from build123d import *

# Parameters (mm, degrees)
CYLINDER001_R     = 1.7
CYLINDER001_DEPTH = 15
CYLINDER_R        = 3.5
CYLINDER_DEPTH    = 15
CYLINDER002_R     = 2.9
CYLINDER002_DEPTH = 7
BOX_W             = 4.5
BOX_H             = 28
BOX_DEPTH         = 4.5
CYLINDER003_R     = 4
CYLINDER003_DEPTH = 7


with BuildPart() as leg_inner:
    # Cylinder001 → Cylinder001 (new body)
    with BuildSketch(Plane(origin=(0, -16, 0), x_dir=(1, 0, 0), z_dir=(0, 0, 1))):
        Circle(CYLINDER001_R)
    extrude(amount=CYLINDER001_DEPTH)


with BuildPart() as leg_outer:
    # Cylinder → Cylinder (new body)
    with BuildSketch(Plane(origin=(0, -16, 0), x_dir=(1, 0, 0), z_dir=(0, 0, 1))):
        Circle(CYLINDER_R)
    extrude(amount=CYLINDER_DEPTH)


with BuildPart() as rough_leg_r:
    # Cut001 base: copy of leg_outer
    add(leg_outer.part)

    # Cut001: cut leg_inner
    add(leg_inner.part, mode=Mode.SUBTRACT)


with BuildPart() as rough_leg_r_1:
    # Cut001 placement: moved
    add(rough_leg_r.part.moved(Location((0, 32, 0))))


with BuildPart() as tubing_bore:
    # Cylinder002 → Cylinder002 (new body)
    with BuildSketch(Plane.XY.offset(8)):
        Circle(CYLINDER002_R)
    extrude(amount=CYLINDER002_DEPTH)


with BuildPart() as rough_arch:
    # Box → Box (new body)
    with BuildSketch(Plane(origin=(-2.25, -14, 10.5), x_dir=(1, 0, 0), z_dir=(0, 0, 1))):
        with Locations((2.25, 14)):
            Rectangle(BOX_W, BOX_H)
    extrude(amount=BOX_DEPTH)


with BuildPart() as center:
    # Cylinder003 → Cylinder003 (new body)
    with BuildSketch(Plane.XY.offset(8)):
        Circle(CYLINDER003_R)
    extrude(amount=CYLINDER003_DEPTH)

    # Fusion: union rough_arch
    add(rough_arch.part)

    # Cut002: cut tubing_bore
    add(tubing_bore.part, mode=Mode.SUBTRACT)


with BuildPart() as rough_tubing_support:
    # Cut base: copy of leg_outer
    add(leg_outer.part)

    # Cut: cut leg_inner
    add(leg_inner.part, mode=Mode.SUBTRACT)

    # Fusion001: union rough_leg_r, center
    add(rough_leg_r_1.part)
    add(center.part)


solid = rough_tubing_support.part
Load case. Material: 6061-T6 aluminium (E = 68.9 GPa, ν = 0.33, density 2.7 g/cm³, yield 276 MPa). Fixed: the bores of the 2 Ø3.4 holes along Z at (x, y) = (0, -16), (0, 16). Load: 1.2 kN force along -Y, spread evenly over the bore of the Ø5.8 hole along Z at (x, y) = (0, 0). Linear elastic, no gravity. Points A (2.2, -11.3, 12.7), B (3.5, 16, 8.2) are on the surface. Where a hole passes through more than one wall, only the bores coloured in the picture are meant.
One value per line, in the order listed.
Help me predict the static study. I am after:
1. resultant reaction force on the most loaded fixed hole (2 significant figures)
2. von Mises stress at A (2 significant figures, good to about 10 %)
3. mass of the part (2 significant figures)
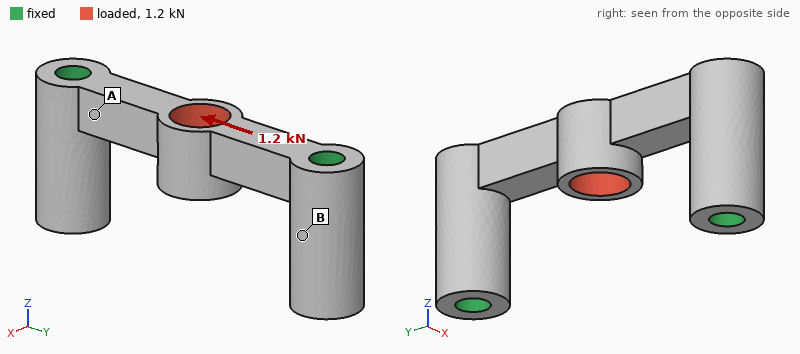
600 N
31 MPa
3.8 g
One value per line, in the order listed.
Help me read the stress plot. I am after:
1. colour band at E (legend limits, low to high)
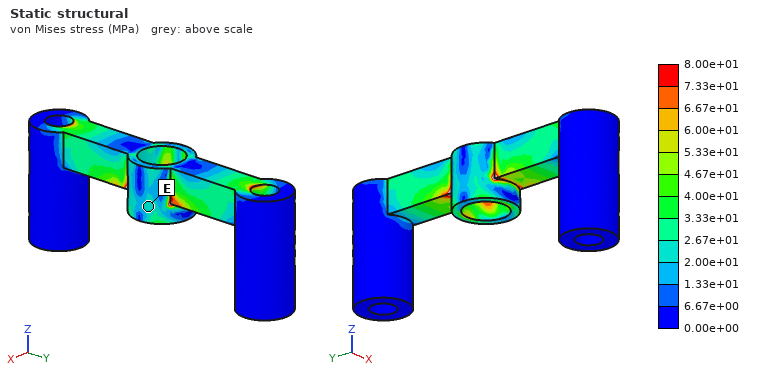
2.00e+01 to 2.67e+01 MPa
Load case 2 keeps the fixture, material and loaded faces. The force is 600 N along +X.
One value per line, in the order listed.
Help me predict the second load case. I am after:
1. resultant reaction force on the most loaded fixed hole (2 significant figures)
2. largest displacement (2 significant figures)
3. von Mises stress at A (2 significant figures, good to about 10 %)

300 N
51 µm
88 MPa
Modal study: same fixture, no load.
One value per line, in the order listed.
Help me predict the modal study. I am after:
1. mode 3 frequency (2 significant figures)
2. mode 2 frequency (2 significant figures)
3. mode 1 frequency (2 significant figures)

34 kHz
23 kHz
22 kHz
